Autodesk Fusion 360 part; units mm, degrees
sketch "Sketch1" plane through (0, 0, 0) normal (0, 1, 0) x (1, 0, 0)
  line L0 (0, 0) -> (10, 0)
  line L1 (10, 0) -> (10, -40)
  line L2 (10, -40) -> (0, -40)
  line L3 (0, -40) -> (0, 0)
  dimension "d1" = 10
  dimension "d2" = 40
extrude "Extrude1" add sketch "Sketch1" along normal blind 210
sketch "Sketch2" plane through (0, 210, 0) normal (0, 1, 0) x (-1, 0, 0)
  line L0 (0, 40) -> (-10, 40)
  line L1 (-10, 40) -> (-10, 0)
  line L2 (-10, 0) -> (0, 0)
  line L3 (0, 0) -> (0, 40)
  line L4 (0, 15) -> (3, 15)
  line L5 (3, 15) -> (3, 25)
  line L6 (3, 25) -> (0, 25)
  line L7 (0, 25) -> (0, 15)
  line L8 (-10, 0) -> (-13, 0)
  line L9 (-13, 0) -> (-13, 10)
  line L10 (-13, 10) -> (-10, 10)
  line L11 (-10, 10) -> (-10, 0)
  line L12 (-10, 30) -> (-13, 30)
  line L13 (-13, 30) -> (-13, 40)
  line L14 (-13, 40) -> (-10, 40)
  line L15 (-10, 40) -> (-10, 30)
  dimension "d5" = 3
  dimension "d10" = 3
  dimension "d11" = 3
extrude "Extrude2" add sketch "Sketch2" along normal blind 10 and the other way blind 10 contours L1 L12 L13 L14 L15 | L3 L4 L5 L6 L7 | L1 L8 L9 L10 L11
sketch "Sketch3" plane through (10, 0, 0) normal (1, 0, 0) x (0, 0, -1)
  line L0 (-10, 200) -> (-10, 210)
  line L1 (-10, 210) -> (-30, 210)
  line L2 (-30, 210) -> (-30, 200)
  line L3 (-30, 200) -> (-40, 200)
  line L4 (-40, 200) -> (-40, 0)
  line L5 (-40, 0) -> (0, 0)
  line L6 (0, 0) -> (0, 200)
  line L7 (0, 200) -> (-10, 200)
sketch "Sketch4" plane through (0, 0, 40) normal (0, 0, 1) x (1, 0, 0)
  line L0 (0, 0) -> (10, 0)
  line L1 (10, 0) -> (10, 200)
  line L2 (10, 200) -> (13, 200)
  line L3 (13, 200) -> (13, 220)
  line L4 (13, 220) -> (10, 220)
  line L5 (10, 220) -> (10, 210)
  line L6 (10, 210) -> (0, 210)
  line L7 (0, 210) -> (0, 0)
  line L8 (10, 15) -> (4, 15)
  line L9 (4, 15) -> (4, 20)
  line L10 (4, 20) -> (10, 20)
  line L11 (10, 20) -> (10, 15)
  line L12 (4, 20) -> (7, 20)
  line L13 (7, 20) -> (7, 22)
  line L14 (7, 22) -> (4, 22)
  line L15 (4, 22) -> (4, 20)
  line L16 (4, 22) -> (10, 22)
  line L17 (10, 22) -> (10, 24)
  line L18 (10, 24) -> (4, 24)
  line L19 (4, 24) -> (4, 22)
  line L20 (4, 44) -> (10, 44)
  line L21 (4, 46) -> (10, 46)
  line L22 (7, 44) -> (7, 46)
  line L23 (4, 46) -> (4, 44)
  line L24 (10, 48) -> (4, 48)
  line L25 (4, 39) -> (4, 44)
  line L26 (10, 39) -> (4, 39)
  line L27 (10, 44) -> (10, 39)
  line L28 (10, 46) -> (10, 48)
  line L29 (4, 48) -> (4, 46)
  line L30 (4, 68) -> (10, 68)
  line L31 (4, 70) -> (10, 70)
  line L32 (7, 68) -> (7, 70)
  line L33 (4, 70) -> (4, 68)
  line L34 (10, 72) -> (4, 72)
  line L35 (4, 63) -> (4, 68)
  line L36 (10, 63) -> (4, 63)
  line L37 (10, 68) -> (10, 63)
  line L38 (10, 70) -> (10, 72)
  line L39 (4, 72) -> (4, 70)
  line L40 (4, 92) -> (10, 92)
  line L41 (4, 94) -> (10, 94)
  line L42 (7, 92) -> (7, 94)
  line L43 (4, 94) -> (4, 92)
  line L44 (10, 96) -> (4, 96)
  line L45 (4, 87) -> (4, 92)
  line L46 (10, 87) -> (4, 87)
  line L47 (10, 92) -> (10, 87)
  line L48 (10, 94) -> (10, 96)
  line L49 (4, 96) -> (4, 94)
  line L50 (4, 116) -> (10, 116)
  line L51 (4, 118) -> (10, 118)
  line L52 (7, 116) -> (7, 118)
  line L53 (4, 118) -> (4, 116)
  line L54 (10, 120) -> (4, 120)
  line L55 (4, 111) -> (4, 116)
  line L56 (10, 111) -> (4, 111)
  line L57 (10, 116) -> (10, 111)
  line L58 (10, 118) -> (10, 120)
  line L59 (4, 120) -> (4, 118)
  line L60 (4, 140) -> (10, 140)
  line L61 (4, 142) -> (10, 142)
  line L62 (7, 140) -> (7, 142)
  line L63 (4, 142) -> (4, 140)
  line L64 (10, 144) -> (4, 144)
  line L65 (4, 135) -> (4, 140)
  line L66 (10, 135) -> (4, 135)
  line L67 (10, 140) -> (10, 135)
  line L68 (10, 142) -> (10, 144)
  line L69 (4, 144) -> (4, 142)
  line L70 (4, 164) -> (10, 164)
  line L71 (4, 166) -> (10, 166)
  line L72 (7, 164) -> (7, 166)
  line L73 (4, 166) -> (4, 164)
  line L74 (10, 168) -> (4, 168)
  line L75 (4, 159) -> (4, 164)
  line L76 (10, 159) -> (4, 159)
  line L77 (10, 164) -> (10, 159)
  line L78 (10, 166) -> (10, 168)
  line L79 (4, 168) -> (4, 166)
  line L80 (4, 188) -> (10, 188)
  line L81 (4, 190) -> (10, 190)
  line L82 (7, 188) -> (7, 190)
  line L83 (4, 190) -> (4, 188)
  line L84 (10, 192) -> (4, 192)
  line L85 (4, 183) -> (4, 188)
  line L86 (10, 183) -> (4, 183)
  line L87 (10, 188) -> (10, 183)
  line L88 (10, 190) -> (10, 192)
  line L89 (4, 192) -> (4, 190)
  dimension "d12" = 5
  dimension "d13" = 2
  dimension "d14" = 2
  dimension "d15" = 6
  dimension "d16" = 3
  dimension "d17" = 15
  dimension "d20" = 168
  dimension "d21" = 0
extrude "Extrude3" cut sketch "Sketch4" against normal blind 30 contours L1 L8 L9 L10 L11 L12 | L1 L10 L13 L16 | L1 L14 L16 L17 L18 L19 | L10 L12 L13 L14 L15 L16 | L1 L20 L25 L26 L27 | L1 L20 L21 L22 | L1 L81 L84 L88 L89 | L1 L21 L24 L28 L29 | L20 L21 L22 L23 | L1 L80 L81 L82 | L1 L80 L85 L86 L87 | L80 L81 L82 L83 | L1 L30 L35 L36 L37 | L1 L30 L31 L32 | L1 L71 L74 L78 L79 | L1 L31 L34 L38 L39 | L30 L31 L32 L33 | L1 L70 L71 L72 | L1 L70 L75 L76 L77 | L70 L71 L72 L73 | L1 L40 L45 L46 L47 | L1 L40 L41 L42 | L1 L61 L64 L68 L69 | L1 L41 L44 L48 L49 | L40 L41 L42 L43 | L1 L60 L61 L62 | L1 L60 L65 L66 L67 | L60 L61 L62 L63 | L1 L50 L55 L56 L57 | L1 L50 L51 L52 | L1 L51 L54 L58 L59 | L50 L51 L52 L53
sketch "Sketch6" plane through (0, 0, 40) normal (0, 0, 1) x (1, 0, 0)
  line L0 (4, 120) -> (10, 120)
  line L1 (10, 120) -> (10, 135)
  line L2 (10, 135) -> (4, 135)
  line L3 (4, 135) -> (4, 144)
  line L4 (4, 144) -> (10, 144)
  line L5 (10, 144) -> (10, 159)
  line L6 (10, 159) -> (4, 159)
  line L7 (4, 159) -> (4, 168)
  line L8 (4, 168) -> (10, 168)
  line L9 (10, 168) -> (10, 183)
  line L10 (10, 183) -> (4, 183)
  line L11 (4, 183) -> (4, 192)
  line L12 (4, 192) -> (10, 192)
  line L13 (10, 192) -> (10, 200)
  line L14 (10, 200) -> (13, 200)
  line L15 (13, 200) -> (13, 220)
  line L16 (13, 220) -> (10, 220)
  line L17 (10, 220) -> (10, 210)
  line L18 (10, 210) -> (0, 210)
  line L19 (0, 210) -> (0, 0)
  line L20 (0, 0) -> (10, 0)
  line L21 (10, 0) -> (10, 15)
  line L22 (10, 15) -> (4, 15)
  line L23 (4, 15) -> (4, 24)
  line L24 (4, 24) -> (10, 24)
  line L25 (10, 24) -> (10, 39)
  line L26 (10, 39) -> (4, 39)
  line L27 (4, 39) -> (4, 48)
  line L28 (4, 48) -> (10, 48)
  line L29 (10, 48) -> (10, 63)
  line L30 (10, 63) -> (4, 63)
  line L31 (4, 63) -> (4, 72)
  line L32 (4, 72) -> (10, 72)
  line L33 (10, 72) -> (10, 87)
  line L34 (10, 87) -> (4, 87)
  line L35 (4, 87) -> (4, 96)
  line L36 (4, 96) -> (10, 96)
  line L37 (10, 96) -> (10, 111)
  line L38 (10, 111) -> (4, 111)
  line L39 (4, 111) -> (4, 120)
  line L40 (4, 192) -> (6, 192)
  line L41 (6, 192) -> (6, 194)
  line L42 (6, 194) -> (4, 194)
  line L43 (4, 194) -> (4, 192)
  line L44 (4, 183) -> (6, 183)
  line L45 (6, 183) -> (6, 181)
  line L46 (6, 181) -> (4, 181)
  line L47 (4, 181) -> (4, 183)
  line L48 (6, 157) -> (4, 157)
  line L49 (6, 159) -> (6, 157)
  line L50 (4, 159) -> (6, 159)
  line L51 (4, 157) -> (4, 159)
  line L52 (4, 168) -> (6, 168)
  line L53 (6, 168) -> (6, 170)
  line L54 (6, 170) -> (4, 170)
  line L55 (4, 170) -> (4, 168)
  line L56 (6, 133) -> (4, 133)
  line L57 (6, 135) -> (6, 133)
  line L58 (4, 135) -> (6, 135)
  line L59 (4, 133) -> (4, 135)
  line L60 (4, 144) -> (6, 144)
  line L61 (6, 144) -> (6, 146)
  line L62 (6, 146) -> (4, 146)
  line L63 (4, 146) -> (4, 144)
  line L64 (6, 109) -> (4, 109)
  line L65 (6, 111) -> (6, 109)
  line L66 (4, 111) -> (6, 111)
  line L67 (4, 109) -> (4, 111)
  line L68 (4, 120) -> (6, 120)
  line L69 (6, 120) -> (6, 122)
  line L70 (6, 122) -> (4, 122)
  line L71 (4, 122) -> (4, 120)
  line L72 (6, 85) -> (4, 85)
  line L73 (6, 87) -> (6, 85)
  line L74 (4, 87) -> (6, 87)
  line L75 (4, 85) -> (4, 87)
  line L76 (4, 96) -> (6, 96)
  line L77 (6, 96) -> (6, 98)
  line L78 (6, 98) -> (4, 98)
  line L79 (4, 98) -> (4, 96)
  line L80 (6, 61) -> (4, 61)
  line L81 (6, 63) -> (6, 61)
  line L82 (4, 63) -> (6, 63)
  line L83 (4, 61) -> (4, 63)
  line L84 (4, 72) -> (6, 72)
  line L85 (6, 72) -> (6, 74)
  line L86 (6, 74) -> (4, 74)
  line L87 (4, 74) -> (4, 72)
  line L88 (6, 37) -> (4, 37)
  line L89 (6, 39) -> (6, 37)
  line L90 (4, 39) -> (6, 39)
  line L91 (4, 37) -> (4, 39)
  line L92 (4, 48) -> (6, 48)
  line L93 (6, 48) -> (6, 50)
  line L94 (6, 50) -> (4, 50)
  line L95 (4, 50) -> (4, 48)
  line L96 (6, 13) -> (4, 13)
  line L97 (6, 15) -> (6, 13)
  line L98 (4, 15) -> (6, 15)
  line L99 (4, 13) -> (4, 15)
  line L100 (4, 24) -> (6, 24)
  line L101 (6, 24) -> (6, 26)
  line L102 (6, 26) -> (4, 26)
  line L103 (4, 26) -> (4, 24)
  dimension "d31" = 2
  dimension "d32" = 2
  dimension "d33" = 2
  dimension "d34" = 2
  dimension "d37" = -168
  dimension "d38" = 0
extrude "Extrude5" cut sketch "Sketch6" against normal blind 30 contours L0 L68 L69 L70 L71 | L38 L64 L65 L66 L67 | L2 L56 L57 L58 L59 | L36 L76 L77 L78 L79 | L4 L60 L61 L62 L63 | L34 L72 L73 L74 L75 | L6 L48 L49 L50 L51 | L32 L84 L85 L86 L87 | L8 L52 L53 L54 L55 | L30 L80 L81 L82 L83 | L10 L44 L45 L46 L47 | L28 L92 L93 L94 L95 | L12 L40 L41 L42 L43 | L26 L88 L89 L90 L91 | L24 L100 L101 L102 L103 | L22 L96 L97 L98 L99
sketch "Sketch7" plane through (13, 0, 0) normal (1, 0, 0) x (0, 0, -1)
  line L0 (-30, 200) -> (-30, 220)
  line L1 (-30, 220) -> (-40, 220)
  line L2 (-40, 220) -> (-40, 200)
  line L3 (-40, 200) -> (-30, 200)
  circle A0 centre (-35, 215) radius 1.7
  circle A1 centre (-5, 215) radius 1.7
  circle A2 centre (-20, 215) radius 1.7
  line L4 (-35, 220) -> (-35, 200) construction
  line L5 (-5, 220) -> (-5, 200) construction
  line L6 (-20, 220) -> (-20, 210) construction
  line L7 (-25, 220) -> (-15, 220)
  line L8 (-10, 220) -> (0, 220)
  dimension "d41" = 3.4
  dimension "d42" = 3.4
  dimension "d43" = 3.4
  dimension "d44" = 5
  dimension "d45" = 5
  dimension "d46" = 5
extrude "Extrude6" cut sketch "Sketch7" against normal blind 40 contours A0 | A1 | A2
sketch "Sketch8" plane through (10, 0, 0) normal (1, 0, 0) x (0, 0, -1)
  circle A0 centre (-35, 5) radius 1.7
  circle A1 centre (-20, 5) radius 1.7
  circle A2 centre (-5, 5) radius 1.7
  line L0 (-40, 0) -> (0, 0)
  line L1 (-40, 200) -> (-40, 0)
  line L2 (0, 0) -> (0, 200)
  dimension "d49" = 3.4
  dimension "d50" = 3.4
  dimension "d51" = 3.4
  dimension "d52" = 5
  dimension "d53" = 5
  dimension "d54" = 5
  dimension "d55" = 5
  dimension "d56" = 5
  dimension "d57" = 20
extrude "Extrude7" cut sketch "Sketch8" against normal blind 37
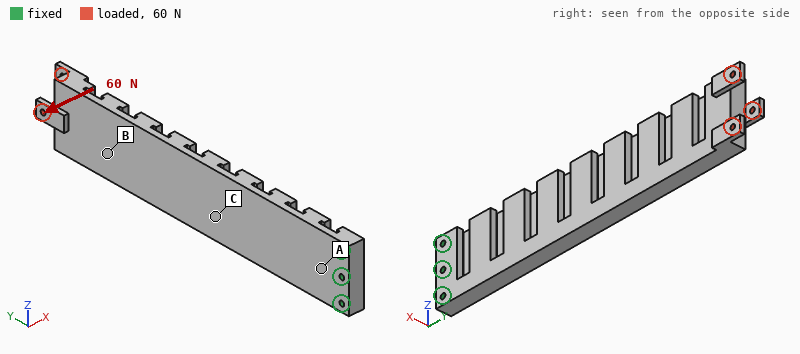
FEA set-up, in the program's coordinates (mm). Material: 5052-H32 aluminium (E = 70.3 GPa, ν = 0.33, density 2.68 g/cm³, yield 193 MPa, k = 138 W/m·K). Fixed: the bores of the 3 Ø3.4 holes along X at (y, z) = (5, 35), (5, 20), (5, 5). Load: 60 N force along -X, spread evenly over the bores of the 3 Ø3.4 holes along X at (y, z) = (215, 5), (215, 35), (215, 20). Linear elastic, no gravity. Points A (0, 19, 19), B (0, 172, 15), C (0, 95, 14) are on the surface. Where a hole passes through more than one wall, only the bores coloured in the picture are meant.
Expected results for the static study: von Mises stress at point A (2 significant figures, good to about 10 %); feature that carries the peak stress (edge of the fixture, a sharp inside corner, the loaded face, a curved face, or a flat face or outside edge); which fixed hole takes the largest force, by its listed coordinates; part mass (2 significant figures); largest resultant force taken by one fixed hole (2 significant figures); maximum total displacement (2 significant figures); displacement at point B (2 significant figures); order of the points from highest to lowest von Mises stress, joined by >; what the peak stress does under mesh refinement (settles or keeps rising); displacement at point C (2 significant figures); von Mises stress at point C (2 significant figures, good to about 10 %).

32 MPa
edge of the fixture
(5, 20)
190 g
300 N
2.1 mm
1.4 mm
A > C > B
keeps rising
0.48 mm
22 MPa
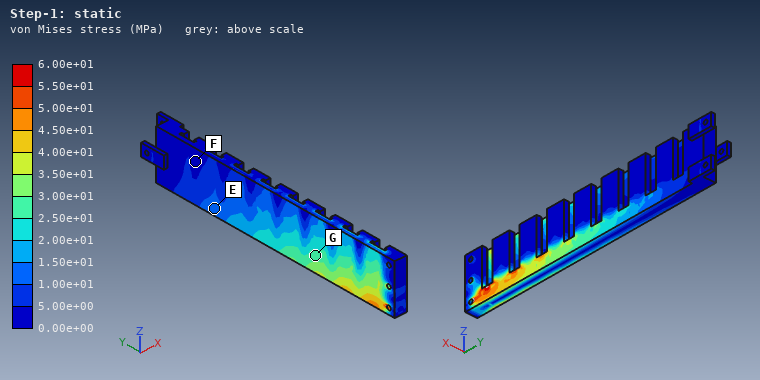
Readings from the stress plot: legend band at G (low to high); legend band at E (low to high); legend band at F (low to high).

2.50e+01 to 3.00e+01 MPa
1.00e+01 to 1.50e+01 MPa
0.00e+00 to 5.00e+00 MPa
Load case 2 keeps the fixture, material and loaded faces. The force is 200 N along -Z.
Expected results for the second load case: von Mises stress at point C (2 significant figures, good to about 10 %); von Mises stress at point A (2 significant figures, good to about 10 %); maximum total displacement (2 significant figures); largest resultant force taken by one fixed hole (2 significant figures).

9.7 MPa
8.3 MPa
0.79 mm
1.4 kN
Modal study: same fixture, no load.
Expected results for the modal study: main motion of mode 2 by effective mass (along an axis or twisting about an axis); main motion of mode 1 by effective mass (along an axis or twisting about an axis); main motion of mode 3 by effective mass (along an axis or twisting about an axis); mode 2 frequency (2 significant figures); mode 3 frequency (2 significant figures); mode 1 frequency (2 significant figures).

along Z
along X
along X
620 Hz
780 Hz
130 Hz
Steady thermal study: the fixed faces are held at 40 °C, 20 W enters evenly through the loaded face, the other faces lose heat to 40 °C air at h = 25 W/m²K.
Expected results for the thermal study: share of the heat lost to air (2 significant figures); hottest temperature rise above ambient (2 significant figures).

74 %
66 K
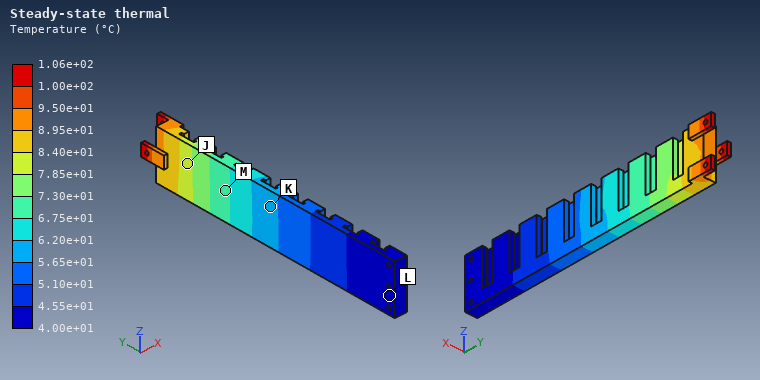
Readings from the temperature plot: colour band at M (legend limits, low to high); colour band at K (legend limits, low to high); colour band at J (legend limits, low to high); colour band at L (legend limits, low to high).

6.75e+01 to 7.30e+01 °C
5.65e+01 to 6.20e+01 °C
7.85e+01 to 8.40e+01 °C
4.00e+01 to 4.55e+01 °C
